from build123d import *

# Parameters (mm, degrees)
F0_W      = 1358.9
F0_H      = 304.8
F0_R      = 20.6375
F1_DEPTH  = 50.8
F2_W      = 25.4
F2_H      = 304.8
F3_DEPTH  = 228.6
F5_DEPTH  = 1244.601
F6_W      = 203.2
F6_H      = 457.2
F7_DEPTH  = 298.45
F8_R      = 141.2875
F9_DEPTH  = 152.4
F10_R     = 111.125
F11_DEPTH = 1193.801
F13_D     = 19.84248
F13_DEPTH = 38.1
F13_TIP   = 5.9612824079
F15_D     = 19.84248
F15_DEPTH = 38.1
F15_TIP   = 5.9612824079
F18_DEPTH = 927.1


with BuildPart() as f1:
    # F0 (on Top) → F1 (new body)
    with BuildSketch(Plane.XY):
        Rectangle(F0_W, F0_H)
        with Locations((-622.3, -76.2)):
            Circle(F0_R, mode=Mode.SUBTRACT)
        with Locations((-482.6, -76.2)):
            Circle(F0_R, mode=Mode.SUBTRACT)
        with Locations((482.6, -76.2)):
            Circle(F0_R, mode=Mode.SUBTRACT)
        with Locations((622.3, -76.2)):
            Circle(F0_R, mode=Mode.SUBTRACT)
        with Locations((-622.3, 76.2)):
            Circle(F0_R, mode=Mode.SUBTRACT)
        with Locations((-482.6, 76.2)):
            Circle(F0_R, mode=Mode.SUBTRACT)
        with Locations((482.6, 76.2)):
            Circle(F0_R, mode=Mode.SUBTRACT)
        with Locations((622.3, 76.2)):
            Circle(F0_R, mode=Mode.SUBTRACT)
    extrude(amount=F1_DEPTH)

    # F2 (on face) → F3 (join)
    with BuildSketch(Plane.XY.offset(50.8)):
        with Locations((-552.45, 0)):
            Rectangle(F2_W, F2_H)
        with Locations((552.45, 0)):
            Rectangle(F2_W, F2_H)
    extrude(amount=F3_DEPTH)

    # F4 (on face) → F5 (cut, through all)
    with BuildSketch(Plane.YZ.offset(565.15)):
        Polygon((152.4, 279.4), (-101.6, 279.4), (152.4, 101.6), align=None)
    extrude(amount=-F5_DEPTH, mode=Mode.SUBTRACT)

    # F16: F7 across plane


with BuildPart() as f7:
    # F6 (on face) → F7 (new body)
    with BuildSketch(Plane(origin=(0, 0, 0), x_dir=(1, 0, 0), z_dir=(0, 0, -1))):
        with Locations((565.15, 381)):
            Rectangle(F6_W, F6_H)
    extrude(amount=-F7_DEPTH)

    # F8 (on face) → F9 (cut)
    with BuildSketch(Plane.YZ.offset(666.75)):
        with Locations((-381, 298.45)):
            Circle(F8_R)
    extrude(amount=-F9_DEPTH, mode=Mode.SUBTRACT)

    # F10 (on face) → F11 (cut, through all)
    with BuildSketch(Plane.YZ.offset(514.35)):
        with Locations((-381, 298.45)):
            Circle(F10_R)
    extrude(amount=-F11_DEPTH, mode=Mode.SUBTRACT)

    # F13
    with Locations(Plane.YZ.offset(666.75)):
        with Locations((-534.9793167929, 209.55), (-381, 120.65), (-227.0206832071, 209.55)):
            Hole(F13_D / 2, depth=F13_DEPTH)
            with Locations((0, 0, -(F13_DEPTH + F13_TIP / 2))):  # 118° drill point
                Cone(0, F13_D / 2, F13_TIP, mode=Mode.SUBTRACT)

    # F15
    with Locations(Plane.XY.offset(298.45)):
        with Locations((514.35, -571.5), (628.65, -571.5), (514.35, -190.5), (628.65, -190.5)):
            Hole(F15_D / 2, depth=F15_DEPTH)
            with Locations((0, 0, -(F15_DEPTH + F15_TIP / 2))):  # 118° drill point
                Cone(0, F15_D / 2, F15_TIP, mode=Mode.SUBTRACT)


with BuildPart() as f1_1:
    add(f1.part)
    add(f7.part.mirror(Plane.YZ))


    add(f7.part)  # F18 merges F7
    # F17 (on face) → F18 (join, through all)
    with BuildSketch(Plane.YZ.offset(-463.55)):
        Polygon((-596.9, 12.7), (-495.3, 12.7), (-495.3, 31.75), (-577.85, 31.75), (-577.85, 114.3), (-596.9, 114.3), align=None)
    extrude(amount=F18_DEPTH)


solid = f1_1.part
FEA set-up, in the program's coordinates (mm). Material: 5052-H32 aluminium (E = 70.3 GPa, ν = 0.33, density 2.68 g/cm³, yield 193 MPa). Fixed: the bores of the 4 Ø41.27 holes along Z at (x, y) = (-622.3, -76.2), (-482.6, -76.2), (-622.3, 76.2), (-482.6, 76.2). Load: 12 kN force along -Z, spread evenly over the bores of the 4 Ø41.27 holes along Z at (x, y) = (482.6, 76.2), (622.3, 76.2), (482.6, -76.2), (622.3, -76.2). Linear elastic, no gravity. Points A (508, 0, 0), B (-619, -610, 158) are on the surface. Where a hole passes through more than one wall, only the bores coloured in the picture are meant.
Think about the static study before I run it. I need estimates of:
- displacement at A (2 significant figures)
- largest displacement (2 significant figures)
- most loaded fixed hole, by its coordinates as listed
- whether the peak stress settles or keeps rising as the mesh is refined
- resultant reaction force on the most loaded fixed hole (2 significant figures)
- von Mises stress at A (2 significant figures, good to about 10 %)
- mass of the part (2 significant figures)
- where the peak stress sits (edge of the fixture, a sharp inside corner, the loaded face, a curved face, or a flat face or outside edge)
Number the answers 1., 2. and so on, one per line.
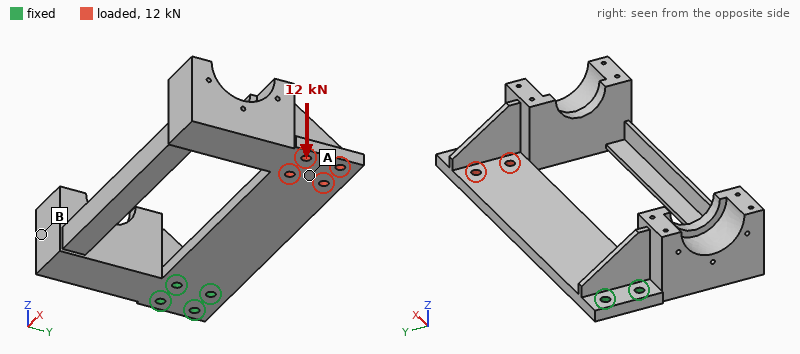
1. 10 mm
2. 14 mm
3. (-482.6, -76.2)
4. keeps rising
5. 39 kN
6. 14 MPa
7. 190 kg
8. edge of the fixture
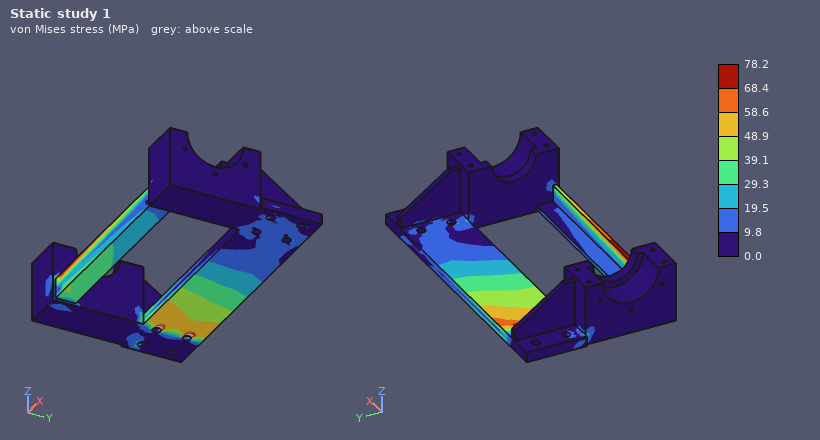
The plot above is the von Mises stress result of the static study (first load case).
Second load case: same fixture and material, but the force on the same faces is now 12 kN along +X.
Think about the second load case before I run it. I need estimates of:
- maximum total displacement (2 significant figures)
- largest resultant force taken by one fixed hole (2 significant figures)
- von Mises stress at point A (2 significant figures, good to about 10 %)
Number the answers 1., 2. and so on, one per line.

1. 14 µm
2. 5.5 kN
3. 0.67 MPa
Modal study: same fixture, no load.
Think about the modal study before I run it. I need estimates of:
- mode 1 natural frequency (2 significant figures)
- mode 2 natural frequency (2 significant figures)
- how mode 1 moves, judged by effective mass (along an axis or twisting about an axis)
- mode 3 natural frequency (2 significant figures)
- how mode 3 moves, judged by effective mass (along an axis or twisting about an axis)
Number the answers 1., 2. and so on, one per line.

1. 19 Hz
2. 57 Hz
3. along Z
4. 100 Hz
5. along Y
